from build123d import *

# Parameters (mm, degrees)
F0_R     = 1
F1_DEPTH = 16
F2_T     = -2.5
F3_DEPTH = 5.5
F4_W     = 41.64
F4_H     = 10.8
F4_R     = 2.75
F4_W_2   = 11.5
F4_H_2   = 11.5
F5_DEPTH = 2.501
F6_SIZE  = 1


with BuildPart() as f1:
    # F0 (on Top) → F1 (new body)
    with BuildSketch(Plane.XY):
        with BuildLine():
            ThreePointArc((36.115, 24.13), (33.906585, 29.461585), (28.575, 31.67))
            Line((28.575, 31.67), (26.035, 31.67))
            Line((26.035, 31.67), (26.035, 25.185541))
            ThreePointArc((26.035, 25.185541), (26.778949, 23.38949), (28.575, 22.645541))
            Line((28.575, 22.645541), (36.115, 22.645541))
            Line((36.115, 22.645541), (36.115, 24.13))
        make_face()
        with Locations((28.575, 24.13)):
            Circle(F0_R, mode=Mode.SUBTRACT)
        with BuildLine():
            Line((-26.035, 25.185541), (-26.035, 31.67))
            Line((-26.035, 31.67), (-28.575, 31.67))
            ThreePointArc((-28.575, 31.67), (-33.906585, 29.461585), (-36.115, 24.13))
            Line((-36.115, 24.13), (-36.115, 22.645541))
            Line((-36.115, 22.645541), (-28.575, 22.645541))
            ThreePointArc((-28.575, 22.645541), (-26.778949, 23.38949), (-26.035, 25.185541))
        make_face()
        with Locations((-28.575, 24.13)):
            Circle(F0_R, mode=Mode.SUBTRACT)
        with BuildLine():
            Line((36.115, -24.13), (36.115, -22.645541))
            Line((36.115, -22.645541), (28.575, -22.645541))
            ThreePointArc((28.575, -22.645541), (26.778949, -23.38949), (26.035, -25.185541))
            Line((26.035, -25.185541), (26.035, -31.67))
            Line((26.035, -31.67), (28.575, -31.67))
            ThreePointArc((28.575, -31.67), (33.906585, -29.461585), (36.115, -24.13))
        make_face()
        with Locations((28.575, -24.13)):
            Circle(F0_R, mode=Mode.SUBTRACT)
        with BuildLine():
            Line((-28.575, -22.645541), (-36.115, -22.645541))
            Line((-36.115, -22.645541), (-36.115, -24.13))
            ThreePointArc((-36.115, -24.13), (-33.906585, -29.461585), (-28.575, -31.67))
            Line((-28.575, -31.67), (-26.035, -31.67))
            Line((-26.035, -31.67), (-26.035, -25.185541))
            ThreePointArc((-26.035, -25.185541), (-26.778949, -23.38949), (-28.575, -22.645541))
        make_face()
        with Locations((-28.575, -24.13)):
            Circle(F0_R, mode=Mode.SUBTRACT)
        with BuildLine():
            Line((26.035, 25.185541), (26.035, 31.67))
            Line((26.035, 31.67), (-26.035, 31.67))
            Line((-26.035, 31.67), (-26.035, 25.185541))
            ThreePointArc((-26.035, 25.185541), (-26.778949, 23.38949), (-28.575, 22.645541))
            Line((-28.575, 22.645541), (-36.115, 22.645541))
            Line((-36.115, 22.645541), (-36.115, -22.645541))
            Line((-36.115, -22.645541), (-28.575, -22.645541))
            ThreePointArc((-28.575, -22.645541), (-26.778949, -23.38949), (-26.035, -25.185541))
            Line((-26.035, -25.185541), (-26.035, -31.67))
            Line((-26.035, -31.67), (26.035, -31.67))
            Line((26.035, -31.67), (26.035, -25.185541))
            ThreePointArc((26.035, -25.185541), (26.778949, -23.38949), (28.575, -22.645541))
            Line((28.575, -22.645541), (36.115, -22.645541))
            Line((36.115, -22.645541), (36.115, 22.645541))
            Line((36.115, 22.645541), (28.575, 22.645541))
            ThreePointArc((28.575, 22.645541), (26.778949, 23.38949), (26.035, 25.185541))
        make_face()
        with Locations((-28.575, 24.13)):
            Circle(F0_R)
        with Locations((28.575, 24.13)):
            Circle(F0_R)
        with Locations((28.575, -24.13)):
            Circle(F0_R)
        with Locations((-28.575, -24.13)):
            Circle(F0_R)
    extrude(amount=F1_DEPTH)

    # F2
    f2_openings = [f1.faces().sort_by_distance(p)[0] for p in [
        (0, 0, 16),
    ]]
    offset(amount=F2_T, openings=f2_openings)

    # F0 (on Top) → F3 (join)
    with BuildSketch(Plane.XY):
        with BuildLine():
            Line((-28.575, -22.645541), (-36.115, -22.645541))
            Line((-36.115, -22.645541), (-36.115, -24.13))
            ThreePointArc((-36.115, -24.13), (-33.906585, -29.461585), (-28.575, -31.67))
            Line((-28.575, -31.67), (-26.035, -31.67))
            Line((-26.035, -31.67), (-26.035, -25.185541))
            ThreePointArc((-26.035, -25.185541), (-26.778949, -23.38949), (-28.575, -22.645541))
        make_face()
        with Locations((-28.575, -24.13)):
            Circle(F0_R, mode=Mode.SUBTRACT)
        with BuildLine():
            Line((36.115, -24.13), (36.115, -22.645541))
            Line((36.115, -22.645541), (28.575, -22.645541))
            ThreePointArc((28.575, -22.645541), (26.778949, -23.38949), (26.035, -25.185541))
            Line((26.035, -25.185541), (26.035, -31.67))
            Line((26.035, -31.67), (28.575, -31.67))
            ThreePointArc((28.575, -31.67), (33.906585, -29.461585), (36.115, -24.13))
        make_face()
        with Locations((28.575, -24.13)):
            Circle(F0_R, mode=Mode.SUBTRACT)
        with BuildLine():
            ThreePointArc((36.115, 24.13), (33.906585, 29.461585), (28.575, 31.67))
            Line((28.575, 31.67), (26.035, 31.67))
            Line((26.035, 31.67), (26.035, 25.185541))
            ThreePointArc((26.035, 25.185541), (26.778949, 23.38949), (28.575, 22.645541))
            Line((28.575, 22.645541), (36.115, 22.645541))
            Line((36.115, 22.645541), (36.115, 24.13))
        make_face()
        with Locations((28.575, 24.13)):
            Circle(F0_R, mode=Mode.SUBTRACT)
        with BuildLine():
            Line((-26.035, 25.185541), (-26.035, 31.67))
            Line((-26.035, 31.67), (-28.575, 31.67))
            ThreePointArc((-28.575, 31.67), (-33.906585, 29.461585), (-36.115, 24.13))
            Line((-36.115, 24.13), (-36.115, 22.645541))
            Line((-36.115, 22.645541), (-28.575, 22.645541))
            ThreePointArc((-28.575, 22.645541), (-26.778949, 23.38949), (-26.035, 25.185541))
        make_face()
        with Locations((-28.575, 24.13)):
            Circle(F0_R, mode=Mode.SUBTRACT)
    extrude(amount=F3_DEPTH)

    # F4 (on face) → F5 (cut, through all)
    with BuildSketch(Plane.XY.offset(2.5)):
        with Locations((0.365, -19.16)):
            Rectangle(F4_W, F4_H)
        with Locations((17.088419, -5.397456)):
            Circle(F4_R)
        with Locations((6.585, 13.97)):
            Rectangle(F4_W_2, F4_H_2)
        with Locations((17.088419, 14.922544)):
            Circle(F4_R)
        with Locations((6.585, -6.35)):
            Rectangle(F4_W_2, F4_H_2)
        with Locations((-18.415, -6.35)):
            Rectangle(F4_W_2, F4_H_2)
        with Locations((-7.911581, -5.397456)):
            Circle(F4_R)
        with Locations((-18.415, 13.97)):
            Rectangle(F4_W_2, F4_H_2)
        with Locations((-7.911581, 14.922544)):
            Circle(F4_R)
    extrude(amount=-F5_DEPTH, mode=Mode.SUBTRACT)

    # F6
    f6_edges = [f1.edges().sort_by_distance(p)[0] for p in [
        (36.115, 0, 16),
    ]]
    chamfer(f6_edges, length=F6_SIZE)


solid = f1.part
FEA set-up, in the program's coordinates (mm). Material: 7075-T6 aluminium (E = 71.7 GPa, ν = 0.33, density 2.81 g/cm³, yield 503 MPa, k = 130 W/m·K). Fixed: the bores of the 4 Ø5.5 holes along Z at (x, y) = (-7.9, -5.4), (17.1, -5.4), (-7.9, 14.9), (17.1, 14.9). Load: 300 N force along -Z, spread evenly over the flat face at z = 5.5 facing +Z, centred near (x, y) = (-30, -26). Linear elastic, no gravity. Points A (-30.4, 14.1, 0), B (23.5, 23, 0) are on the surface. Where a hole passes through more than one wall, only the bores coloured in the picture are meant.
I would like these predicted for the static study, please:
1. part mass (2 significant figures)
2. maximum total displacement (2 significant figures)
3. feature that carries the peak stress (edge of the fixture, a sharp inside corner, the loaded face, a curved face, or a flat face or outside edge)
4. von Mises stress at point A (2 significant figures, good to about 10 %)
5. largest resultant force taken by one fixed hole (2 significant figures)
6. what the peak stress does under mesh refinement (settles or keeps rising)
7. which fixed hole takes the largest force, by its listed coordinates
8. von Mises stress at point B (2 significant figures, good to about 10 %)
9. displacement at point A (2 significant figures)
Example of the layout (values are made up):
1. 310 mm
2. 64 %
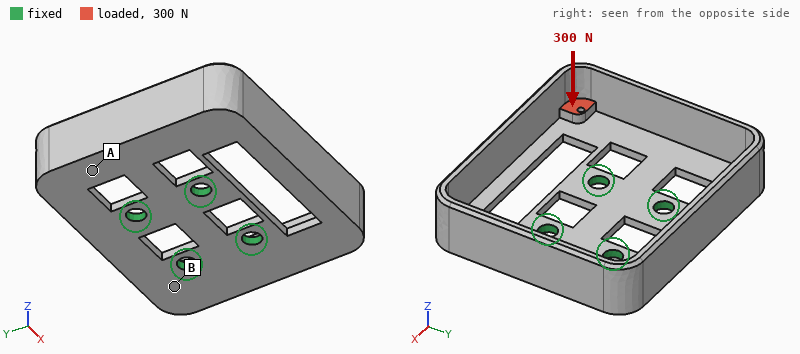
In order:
1. 49 g
2. 0.90 mm
3. a sharp inside corner
4. 79 MPa
5. 340 N
6. keeps rising
7. (-7.9, -5.4)
8. 24 MPa
9. 0.14 mm
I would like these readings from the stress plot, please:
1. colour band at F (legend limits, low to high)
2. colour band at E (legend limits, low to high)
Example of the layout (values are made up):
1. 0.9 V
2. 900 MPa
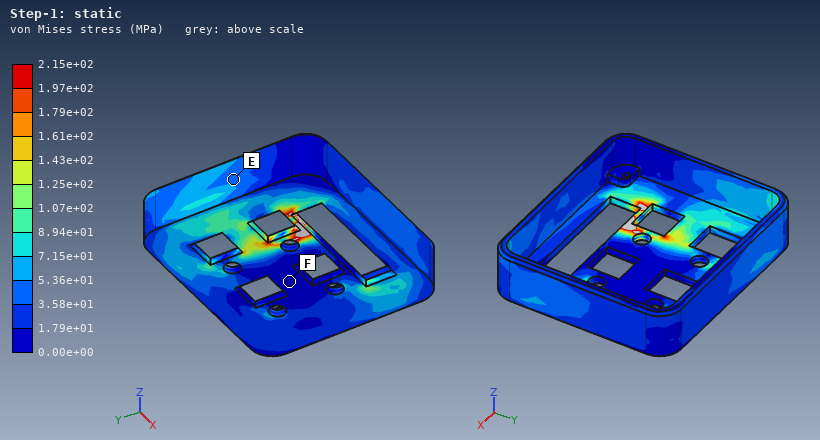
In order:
1. 0.00e+00 to 1.79e+01 MPa
2. 3.58e+01 to 5.36e+01 MPa
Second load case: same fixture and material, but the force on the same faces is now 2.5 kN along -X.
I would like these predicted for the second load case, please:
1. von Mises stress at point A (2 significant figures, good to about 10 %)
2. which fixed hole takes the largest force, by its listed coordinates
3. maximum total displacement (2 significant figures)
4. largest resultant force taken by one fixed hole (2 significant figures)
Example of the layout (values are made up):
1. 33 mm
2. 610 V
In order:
1. 89 MPa
2. (17.1, -5.4)
3. 0.68 mm
4. 2.4 kN
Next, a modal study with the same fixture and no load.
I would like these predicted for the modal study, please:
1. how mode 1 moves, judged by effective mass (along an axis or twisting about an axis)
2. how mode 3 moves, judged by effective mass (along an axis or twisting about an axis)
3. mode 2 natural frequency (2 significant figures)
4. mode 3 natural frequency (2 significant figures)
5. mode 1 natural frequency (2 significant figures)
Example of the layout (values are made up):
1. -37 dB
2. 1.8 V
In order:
1. along Z
2. along Z
3. 2100 Hz
4. 2200 Hz
5. 1100 Hz
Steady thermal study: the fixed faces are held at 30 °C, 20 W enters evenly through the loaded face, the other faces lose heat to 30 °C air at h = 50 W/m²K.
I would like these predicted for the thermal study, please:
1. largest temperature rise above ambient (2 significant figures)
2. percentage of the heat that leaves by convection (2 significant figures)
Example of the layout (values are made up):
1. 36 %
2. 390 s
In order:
1. 64 K
2. 51 %
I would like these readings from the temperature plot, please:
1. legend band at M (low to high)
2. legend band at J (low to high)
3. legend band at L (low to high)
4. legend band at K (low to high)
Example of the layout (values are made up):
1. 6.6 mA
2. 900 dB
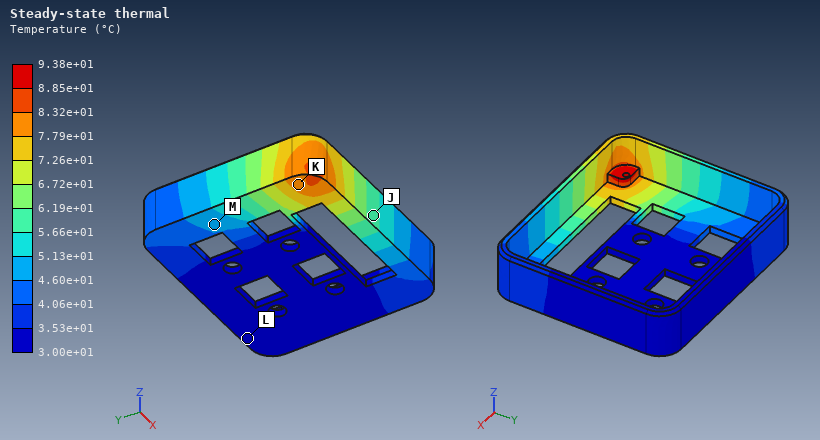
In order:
1. 4.60e+01 to 5.13e+01 °C
2. 5.66e+01 to 6.19e+01 °C
3. 3.00e+01 to 3.53e+01 °C
4. 7.79e+01 to 8.32e+01 °C
